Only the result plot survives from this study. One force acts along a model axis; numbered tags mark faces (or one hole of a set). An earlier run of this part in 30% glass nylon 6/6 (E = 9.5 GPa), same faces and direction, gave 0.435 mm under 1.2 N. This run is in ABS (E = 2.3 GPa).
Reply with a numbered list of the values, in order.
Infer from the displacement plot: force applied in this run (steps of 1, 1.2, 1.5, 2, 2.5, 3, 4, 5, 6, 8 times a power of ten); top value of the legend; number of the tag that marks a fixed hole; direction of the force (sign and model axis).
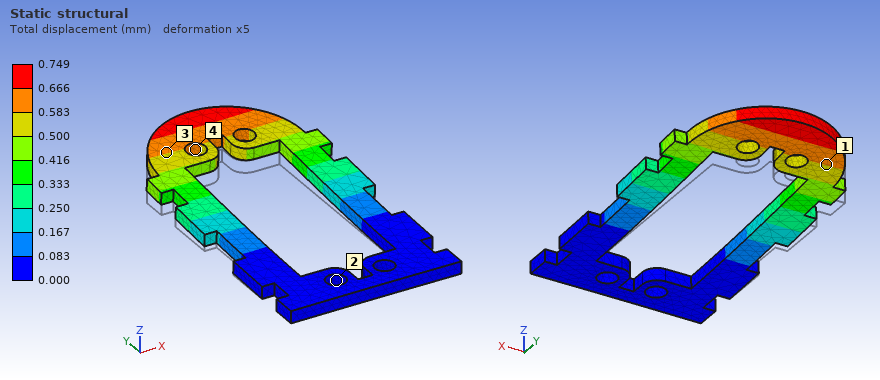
1. 0.5 N
2. 0.749 mm
3. 2
4. +Z
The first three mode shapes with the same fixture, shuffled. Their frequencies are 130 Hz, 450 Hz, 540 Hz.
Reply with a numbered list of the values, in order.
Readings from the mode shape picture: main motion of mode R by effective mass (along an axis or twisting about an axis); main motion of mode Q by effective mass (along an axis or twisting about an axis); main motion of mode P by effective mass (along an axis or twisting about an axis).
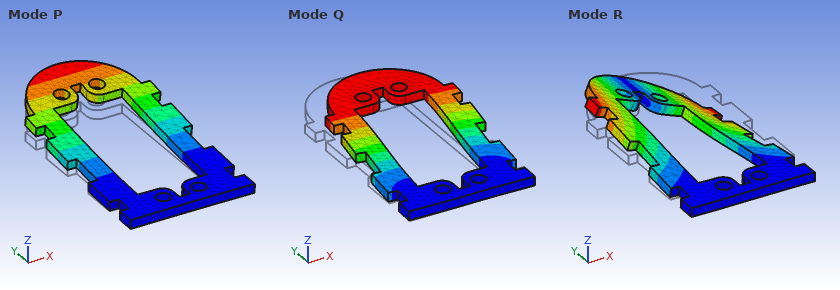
1. twisting about Y
2. along X
3. along Z
